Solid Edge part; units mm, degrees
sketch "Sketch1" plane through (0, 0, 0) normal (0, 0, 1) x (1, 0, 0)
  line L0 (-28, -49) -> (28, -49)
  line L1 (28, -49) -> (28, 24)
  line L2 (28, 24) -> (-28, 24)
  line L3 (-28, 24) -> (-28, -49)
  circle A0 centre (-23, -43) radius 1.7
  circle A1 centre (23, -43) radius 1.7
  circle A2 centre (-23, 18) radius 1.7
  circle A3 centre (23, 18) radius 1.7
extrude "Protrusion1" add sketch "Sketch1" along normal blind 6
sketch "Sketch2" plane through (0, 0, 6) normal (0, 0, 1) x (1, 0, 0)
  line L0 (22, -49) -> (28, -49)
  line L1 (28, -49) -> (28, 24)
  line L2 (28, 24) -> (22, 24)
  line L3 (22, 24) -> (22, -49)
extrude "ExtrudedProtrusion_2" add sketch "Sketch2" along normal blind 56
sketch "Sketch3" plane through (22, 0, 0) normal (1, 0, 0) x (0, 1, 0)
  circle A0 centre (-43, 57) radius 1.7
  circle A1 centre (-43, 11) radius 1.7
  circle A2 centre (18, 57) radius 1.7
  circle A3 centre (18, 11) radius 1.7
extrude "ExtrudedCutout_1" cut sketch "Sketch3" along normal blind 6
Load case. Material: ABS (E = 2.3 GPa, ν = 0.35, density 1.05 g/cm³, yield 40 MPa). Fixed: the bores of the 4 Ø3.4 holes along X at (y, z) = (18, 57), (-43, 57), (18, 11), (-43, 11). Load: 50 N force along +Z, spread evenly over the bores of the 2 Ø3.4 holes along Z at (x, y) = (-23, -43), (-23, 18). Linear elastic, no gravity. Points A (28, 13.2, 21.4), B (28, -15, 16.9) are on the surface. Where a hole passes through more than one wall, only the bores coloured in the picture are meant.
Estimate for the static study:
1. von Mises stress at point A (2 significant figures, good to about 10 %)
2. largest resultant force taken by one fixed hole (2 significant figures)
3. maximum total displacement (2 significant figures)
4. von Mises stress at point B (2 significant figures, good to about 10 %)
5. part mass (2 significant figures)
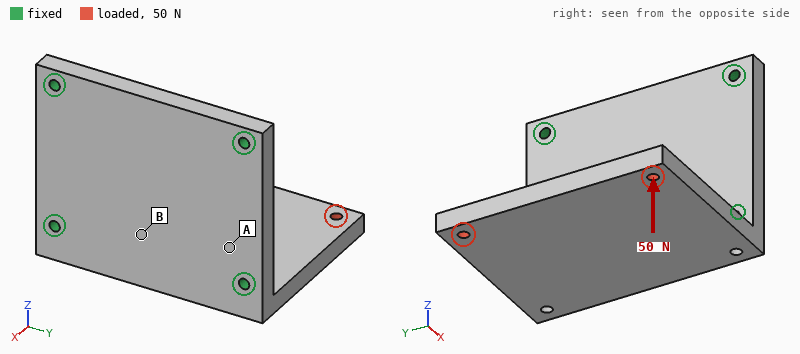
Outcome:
0.95 MPa
19 N
1.1 mm
2.4 MPa
51 g
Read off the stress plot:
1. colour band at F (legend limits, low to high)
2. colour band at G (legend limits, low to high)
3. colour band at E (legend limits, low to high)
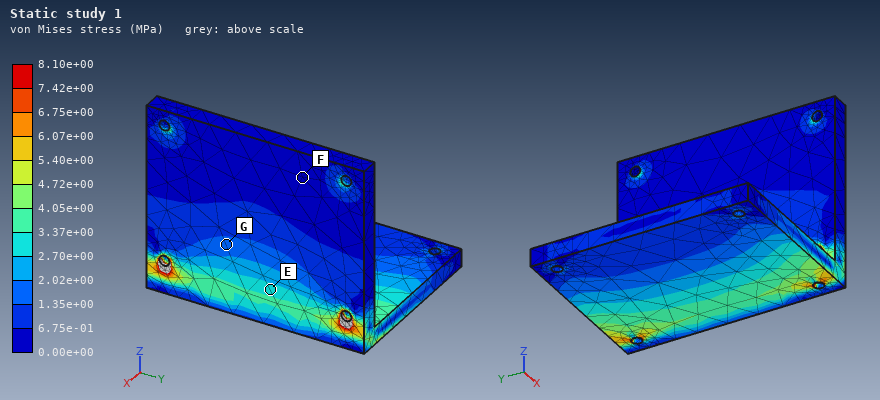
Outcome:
0.00e+00 to 6.75e-01 MPa
1.35e+00 to 2.02e+00 MPa
2.70e+00 to 3.37e+00 MPa
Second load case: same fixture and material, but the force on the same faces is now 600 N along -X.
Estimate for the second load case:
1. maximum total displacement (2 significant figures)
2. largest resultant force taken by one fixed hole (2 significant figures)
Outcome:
0.67 mm
320 N
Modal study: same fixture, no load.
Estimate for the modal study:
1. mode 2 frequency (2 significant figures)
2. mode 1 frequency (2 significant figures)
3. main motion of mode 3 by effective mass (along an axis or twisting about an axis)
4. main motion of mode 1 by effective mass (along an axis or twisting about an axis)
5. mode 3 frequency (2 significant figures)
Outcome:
870 Hz
390 Hz
along Y
along Z
1900 Hz
